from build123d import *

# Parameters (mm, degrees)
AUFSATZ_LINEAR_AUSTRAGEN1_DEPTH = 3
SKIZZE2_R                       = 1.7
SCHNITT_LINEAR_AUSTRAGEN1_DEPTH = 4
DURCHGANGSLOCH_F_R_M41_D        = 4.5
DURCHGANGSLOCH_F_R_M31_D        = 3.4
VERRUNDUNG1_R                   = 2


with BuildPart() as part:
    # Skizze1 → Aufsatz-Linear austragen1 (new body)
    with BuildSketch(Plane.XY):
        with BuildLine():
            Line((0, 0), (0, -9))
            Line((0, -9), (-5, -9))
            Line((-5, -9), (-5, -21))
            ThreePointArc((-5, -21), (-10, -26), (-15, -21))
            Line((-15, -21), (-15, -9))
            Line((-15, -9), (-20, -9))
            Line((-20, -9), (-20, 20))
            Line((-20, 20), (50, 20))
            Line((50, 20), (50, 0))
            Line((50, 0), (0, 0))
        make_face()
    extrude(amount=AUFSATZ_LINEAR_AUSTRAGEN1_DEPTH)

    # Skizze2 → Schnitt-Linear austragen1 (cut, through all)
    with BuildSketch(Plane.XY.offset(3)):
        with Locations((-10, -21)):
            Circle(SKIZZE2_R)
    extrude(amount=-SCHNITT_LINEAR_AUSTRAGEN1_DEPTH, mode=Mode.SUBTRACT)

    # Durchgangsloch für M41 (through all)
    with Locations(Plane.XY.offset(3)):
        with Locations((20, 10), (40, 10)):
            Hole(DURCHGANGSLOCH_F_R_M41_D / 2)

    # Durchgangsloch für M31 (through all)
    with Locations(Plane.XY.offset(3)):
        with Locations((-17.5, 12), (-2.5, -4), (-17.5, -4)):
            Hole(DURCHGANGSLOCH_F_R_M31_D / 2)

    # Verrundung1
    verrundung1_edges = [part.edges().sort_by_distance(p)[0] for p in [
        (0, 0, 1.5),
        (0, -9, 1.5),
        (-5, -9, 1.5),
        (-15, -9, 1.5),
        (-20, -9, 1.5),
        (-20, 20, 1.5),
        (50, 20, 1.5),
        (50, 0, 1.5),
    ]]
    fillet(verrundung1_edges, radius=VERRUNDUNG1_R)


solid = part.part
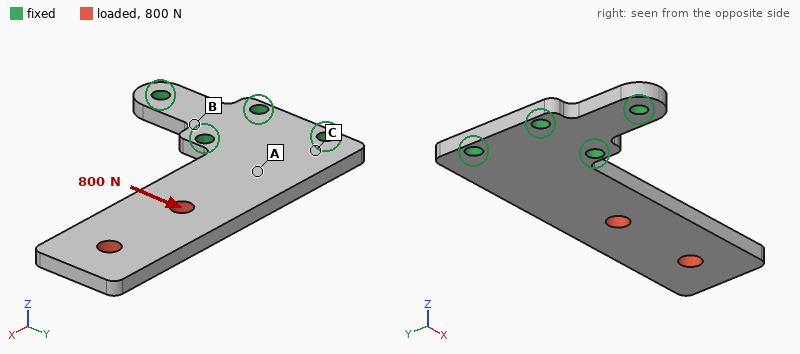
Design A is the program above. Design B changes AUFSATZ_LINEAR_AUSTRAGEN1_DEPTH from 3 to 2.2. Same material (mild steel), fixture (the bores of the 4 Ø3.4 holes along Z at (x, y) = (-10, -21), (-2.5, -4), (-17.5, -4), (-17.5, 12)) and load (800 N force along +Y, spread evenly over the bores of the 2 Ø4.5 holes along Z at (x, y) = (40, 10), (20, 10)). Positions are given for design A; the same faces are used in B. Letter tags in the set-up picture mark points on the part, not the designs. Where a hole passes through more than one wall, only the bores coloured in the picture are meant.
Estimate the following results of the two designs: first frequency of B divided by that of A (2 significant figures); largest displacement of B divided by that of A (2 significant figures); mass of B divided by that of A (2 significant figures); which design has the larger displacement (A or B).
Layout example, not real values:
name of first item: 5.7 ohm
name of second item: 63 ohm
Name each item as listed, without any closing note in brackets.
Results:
first frequency of B divided by that of A: 0.74
largest displacement of B divided by that of A: 1.4
mass of B divided by that of A: 0.73
which design has the larger displacement: B
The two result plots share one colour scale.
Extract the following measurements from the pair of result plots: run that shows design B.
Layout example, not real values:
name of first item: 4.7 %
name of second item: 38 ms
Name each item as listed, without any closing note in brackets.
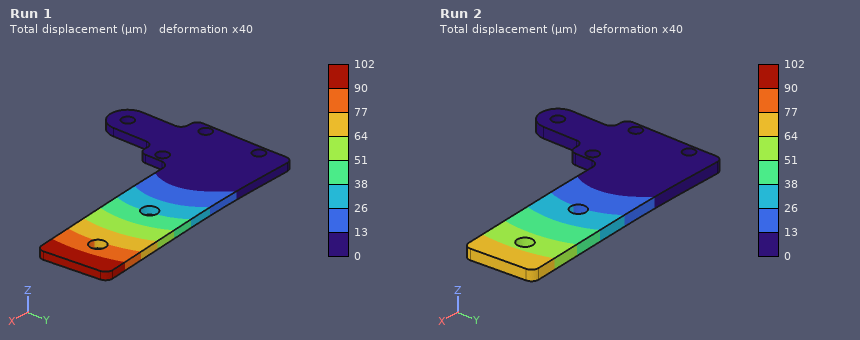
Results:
run that shows design B: Run 1
